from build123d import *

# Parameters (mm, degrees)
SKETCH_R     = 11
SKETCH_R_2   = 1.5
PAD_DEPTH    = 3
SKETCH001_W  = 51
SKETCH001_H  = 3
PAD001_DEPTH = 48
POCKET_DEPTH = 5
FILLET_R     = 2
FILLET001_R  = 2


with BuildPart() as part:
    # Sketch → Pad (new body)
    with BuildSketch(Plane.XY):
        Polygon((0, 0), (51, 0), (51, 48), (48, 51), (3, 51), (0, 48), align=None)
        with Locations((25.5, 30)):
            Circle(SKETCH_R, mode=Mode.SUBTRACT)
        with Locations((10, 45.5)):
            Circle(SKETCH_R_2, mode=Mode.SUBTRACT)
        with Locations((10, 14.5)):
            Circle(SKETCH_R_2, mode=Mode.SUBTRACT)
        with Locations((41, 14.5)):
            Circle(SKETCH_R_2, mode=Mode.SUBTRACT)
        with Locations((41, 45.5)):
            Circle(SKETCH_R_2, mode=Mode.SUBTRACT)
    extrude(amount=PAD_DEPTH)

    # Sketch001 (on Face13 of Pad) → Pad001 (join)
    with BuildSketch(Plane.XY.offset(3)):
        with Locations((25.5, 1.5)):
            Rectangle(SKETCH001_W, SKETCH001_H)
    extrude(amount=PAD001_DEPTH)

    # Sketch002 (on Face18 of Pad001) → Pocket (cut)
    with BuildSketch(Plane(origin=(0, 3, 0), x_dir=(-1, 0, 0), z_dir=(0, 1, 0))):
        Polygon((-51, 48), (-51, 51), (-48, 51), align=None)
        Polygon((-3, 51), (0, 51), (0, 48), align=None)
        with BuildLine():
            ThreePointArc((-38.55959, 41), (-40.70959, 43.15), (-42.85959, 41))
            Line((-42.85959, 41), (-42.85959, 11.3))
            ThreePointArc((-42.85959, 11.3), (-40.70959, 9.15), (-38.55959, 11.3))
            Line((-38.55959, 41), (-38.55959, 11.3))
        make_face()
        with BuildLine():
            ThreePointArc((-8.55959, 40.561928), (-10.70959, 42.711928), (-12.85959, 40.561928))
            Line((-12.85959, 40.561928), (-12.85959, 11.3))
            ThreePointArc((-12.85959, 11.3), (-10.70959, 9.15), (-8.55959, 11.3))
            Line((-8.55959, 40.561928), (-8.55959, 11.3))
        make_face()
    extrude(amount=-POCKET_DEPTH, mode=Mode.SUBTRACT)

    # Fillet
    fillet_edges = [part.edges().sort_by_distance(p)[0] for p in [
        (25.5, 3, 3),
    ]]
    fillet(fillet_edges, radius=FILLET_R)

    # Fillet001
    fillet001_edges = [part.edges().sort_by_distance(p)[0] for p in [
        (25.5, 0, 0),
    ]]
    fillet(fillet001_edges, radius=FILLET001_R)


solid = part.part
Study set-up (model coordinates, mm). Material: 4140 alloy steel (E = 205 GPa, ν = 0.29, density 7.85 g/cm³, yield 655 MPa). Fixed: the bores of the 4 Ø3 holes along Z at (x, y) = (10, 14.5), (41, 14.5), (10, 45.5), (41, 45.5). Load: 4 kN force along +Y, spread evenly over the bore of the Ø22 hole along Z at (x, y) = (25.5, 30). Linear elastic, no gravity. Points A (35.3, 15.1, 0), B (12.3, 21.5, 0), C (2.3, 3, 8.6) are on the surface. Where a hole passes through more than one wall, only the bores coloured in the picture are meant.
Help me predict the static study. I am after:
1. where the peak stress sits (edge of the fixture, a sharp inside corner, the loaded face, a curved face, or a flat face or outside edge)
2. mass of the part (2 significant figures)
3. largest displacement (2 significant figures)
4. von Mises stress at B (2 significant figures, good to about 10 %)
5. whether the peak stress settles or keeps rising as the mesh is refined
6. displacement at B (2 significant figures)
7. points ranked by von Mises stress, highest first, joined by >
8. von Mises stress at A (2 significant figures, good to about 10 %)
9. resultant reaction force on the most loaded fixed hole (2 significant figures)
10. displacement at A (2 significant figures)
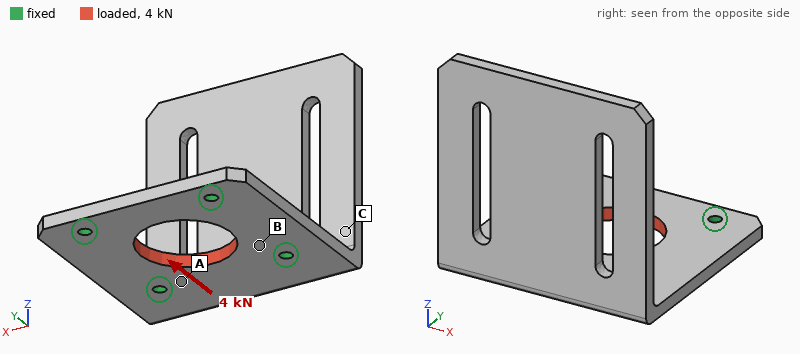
edge of the fixture
100 g
4.1 µm
27 MPa
keeps rising
0.93 µm
B > A > C
17 MPa
1.0 kN
1.1 µm
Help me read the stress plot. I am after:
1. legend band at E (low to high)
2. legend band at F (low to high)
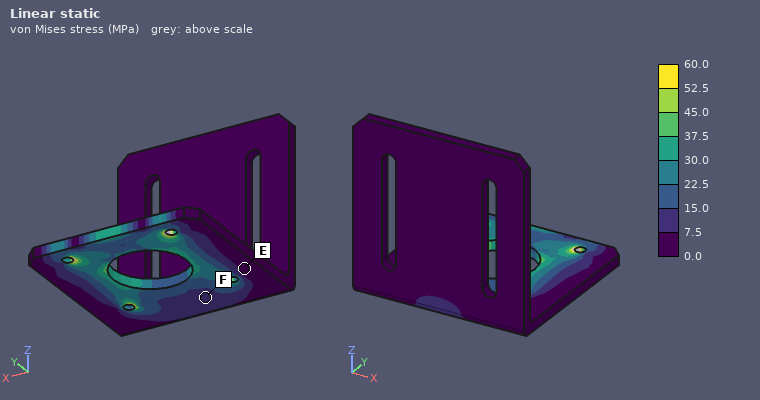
0.0 to 7.5 MPa
7.5 to 15.0 MPa
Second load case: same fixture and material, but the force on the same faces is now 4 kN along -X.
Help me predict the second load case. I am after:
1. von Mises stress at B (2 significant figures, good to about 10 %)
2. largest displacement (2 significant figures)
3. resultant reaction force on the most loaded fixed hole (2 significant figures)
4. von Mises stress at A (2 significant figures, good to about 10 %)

22 MPa
3.1 µm
1.0 kN
26 MPa
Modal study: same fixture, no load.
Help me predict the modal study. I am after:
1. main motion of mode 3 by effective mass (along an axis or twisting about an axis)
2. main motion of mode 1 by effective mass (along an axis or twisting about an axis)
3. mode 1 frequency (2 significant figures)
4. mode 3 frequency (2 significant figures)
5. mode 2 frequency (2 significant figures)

along X
along Y
740 Hz
2700 Hz
1900 Hz
